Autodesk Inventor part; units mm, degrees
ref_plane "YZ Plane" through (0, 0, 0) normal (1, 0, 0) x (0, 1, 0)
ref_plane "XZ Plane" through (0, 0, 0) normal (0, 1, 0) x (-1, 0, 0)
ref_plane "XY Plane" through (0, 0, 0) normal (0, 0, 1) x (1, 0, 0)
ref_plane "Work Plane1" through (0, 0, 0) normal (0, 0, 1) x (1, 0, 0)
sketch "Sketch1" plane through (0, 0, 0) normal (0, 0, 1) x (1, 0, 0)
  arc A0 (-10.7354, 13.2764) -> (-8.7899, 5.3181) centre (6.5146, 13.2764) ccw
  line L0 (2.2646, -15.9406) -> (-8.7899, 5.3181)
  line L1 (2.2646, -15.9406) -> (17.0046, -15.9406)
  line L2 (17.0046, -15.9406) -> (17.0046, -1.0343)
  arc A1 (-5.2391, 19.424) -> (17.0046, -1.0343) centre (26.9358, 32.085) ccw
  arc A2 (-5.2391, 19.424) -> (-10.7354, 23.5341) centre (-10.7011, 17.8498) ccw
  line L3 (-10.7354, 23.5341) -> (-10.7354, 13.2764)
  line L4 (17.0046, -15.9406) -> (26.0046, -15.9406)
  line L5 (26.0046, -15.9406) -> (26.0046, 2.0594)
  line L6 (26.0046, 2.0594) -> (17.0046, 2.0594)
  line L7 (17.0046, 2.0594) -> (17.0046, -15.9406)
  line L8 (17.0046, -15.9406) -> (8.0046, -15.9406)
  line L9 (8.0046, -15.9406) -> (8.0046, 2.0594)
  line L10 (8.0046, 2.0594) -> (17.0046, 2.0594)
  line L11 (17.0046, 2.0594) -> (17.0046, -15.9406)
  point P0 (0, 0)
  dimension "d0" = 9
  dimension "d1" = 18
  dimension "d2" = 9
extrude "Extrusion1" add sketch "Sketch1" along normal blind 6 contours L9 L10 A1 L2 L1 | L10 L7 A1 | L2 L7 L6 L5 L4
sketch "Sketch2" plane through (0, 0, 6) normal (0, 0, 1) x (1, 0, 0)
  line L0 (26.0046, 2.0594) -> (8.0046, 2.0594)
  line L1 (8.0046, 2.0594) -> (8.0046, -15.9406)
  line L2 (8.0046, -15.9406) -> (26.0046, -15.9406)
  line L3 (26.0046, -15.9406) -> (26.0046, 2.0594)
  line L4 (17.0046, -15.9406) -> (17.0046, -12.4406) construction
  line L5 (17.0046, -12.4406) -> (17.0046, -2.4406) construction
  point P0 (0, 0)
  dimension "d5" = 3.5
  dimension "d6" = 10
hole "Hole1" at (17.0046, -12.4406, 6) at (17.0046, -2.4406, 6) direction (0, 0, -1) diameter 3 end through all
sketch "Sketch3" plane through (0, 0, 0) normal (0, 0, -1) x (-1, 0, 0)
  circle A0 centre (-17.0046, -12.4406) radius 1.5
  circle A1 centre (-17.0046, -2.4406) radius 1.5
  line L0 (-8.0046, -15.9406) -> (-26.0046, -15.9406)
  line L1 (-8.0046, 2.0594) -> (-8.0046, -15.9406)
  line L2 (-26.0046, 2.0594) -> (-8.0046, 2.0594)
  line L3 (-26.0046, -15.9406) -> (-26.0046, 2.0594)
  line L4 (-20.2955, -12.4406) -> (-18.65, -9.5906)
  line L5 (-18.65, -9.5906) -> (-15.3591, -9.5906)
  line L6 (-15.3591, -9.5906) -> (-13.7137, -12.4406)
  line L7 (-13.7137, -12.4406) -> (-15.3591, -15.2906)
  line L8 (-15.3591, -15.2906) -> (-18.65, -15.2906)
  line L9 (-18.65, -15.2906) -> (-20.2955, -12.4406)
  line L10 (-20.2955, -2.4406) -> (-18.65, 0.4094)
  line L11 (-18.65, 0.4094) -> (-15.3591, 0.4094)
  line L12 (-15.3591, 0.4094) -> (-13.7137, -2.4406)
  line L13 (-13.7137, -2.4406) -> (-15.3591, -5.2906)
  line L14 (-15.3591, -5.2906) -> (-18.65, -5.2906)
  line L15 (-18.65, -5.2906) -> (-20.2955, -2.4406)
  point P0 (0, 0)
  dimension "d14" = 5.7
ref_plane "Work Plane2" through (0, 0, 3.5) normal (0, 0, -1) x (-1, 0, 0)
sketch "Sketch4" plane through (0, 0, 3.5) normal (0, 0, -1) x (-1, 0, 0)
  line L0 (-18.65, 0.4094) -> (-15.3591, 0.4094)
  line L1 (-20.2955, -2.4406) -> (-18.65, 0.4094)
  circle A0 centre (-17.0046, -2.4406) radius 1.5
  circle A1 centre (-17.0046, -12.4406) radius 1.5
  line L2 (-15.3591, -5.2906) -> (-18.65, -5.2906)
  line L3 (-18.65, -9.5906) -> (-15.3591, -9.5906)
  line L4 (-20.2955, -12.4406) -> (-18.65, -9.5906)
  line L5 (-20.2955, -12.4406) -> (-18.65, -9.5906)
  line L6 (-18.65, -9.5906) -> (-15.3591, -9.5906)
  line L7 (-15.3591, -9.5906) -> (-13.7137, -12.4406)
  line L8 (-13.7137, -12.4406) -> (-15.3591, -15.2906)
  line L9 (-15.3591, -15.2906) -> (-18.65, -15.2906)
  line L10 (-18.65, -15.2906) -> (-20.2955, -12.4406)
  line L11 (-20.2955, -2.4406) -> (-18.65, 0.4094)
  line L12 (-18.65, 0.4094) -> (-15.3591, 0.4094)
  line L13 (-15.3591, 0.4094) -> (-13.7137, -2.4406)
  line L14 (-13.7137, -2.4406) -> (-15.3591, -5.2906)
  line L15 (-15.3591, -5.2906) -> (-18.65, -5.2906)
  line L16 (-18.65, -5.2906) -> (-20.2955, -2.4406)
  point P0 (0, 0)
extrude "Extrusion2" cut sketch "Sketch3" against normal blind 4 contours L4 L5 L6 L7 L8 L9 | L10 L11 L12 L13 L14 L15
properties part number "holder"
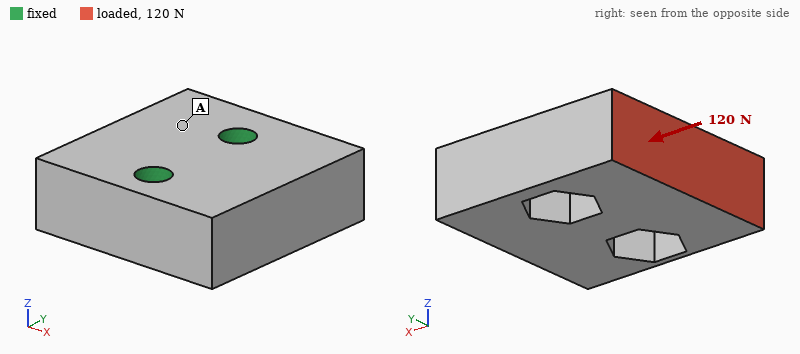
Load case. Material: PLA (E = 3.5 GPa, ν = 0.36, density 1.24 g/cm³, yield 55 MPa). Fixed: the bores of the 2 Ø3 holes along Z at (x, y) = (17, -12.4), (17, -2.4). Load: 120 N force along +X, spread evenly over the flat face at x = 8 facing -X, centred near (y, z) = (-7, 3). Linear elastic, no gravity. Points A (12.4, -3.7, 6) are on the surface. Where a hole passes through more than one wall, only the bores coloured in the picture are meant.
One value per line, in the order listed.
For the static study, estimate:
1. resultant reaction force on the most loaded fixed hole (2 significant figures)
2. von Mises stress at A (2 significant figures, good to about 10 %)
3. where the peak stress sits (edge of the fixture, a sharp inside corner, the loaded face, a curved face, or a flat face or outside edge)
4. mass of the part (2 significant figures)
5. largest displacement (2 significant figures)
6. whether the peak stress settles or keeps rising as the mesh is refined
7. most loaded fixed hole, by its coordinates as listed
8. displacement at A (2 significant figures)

65 N
2.3 MPa
edge of the fixture
2.1 g
42 µm
keeps rising
(17, -2.4)
14 µm
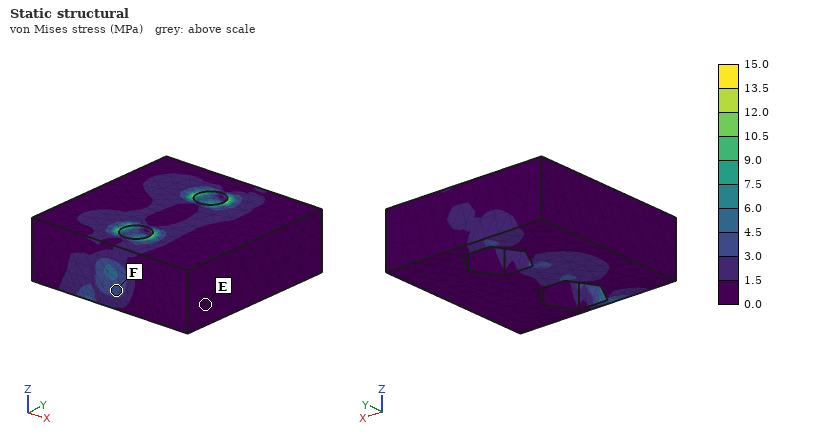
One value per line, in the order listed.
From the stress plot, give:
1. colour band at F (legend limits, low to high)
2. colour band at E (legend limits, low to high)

3.0 to 4.5 MPa
0.0 to 1.5 MPa
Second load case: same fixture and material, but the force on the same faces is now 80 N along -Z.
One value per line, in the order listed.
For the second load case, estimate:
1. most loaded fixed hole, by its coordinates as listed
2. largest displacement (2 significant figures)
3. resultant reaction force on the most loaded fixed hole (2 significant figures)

(17, -2.4)
0.12 mm
44 N
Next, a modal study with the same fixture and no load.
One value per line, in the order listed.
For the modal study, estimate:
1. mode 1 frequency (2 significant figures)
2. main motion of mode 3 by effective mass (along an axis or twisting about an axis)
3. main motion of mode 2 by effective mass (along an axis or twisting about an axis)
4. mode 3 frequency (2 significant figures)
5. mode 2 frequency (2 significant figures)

5100 Hz
along Y
along Z
12 kHz
12 kHz
